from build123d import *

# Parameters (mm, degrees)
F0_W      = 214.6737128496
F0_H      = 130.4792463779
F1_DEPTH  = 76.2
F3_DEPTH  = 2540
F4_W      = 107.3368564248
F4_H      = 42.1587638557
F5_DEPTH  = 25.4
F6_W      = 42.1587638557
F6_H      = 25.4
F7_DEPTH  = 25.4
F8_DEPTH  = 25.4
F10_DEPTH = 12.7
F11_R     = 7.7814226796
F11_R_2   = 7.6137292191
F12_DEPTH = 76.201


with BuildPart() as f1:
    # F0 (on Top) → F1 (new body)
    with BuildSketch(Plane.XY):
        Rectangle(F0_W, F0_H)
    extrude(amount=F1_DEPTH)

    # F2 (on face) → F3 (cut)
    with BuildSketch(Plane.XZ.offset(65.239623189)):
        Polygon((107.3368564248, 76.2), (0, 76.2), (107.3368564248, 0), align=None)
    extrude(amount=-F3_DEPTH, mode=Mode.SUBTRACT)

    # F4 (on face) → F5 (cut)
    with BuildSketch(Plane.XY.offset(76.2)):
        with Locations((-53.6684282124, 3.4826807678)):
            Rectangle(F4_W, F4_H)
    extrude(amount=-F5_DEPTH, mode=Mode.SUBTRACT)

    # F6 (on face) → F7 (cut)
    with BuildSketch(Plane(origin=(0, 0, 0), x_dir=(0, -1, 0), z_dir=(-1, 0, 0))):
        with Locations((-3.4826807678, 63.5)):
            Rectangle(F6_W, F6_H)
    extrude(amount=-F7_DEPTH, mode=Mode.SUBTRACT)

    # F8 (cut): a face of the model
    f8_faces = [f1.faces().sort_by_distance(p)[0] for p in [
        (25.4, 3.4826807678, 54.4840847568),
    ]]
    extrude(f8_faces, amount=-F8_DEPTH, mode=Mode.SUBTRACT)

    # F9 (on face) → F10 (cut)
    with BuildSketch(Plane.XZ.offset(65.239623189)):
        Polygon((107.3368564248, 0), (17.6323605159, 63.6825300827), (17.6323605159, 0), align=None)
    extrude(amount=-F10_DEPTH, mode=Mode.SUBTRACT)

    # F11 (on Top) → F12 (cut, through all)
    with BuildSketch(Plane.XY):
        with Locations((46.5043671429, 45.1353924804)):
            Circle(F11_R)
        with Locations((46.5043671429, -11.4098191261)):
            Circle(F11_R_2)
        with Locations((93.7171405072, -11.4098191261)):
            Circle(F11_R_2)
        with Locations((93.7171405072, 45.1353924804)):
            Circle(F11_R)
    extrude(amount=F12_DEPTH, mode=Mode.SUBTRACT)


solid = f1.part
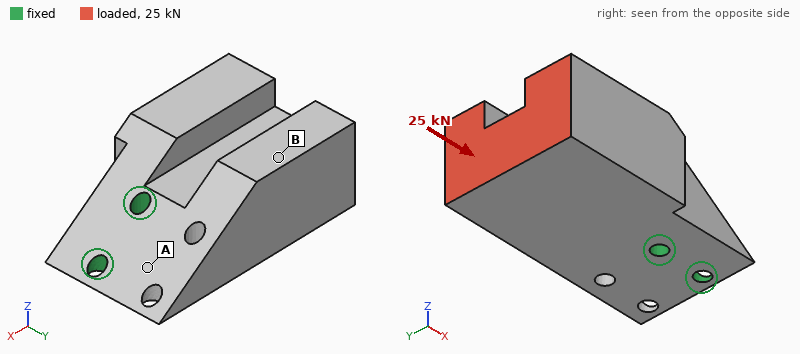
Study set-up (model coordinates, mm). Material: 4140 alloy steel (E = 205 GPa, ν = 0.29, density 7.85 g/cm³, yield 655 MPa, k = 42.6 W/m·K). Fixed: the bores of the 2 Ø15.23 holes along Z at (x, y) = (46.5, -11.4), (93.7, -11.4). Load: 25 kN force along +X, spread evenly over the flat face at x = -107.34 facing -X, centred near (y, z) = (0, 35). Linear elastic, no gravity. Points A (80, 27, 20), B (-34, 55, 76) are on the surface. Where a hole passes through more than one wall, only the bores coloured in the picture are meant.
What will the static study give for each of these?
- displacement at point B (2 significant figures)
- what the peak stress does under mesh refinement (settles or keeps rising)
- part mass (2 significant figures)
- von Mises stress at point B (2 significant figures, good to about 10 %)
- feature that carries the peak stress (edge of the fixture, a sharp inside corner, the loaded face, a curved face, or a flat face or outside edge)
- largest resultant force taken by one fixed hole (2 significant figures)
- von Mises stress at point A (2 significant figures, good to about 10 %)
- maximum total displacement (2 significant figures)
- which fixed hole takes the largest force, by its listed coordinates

13 µm
keeps rising
11 kg
2.3 MPa
edge of the fixture
23 kN
7.3 MPa
19 µm
(46.5, -11.4)
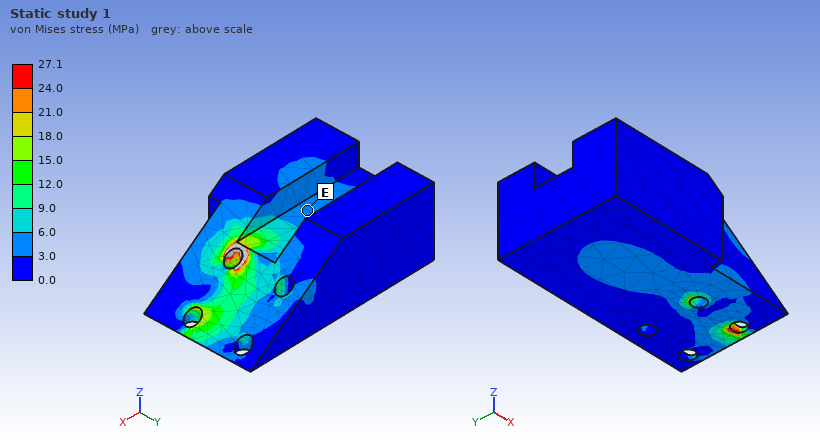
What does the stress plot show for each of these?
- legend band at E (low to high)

3.0 to 6.0 MPa
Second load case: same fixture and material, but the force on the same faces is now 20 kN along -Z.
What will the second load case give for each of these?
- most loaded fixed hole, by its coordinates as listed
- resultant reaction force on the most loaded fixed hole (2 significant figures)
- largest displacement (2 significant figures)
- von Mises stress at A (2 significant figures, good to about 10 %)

(46.5, -11.4)
29 kN
0.15 mm
29 MPa
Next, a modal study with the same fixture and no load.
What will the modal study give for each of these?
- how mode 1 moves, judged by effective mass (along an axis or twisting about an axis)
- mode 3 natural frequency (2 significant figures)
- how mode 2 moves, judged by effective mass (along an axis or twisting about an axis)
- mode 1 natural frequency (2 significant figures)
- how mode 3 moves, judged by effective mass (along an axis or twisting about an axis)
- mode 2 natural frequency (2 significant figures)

along Z
2000 Hz
along Y
1000 Hz
twisting about X
1100 Hz
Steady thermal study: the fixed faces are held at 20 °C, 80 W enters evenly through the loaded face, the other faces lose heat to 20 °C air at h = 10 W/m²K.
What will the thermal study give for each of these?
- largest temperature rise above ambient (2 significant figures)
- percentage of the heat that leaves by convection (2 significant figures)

38 K
21 %
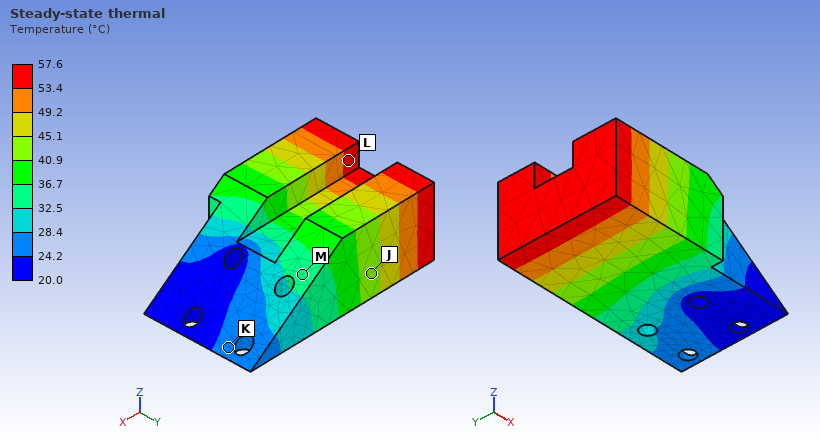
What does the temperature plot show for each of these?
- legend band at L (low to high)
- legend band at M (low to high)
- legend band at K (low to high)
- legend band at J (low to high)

53.4 to 57.6 °C
32.5 to 36.7 °C
24.2 to 28.4 °C
40.9 to 45.1 °C
